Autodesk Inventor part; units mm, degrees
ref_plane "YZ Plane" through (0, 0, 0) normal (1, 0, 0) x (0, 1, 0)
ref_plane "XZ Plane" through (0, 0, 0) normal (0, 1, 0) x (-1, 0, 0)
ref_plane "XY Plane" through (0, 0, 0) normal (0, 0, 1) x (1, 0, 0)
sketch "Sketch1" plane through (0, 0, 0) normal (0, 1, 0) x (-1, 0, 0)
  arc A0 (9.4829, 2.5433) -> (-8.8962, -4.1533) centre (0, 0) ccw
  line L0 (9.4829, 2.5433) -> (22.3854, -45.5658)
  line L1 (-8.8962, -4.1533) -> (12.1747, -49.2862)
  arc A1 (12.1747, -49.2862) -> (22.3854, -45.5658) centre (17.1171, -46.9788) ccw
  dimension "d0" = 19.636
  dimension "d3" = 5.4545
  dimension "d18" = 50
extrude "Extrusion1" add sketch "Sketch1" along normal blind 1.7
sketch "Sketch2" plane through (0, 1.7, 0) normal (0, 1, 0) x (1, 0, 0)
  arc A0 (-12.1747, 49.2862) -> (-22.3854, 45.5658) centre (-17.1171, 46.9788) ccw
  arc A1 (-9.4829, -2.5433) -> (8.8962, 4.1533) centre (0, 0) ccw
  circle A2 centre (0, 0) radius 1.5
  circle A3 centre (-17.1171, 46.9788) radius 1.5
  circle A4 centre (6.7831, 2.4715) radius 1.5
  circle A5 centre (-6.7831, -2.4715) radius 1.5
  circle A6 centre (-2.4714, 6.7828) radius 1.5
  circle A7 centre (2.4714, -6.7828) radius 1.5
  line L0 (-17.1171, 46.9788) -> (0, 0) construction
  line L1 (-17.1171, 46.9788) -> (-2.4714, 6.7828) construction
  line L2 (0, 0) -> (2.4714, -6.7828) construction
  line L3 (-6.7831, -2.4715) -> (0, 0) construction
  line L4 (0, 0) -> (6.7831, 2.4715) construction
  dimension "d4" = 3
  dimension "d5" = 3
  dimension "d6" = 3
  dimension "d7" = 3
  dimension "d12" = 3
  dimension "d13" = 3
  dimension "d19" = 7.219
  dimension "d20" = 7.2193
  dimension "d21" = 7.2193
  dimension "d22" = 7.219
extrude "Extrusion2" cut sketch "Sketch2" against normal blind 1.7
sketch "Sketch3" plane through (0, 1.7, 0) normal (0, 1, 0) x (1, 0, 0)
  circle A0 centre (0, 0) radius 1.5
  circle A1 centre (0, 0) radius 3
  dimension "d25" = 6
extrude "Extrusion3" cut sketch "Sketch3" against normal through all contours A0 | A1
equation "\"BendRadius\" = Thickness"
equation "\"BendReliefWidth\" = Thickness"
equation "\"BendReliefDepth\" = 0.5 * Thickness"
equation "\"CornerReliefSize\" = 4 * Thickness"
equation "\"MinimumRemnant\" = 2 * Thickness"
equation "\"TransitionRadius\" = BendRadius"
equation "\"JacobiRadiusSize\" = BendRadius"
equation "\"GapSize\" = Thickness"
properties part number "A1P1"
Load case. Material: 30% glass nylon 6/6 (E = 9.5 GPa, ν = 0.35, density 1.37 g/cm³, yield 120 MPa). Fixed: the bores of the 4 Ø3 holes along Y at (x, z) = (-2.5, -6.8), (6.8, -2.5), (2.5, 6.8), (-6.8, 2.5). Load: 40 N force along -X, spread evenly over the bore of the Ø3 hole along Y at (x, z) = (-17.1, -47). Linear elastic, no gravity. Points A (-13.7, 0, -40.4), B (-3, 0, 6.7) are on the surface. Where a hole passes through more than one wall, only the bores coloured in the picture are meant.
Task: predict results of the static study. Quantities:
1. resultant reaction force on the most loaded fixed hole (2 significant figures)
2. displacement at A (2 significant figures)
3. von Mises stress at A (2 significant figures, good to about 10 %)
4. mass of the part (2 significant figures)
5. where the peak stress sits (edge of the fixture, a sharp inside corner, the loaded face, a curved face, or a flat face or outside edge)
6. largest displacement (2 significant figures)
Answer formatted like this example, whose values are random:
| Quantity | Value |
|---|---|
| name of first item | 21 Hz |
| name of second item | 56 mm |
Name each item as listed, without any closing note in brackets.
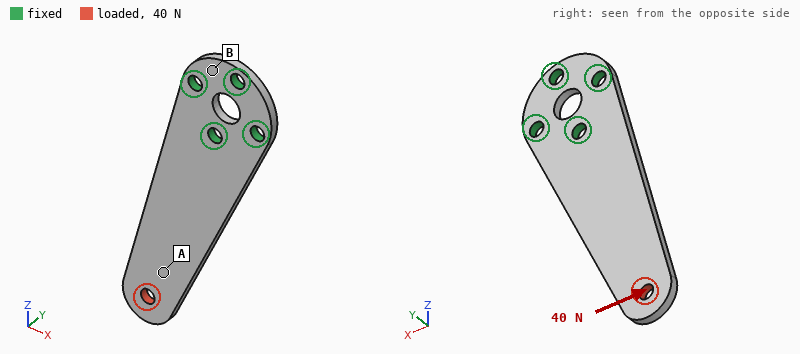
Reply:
| Quantity | Value |
|---|---|
| resultant reaction force on the most loaded fixed hole | 93 N |
| displacement at A | 0.17 mm |
| von Mises stress at A | 4.5 MPa |
| mass of the part | 2.1 g |
| where the peak stress sits | edge of the fixture |
| largest displacement | 0.28 mm |
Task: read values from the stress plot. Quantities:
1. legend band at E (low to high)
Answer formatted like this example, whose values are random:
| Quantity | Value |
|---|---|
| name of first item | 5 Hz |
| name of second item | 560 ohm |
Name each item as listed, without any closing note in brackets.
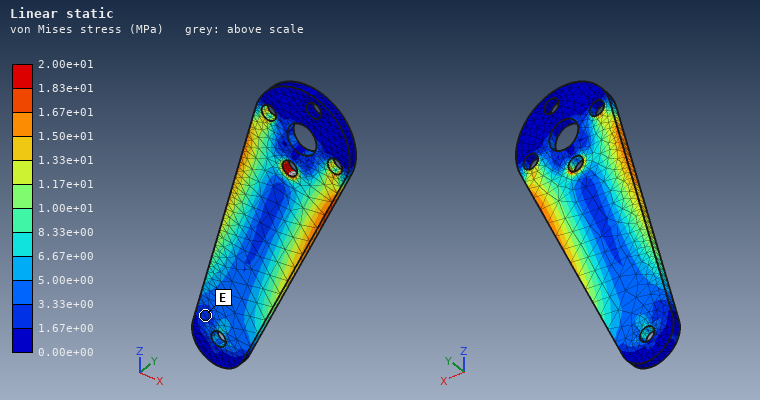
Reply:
| Quantity | Value |
|---|---|
| legend band at E | 1.67e+00 to 3.33e+00 MPa |
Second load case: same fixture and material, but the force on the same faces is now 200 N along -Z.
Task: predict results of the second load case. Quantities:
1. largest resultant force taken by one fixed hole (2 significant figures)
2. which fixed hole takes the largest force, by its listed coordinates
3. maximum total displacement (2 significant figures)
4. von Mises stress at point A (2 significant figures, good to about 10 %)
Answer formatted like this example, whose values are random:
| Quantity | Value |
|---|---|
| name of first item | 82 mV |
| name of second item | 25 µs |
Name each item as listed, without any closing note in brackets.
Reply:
| Quantity | Value |
|---|---|
| largest resultant force taken by one fixed hole | 200 N |
| which fixed hole takes the largest force, by its listed coordinates | (-6.8, 2.5) |
| maximum total displacement | 0.50 mm |
| von Mises stress at point A | 11 MPa |
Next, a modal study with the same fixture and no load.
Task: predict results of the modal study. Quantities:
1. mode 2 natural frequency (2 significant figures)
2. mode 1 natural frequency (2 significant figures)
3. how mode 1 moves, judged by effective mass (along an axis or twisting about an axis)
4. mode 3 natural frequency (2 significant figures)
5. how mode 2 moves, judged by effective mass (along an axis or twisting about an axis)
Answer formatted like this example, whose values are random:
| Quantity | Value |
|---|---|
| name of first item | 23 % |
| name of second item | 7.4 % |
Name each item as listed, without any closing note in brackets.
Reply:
| Quantity | Value |
|---|---|
| mode 2 natural frequency | 2200 Hz |
| mode 1 natural frequency | 410 Hz |
| how mode 1 moves, judged by effective mass | along Y |
| mode 3 natural frequency | 2500 Hz |
| how mode 2 moves, judged by effective mass | along Y |
